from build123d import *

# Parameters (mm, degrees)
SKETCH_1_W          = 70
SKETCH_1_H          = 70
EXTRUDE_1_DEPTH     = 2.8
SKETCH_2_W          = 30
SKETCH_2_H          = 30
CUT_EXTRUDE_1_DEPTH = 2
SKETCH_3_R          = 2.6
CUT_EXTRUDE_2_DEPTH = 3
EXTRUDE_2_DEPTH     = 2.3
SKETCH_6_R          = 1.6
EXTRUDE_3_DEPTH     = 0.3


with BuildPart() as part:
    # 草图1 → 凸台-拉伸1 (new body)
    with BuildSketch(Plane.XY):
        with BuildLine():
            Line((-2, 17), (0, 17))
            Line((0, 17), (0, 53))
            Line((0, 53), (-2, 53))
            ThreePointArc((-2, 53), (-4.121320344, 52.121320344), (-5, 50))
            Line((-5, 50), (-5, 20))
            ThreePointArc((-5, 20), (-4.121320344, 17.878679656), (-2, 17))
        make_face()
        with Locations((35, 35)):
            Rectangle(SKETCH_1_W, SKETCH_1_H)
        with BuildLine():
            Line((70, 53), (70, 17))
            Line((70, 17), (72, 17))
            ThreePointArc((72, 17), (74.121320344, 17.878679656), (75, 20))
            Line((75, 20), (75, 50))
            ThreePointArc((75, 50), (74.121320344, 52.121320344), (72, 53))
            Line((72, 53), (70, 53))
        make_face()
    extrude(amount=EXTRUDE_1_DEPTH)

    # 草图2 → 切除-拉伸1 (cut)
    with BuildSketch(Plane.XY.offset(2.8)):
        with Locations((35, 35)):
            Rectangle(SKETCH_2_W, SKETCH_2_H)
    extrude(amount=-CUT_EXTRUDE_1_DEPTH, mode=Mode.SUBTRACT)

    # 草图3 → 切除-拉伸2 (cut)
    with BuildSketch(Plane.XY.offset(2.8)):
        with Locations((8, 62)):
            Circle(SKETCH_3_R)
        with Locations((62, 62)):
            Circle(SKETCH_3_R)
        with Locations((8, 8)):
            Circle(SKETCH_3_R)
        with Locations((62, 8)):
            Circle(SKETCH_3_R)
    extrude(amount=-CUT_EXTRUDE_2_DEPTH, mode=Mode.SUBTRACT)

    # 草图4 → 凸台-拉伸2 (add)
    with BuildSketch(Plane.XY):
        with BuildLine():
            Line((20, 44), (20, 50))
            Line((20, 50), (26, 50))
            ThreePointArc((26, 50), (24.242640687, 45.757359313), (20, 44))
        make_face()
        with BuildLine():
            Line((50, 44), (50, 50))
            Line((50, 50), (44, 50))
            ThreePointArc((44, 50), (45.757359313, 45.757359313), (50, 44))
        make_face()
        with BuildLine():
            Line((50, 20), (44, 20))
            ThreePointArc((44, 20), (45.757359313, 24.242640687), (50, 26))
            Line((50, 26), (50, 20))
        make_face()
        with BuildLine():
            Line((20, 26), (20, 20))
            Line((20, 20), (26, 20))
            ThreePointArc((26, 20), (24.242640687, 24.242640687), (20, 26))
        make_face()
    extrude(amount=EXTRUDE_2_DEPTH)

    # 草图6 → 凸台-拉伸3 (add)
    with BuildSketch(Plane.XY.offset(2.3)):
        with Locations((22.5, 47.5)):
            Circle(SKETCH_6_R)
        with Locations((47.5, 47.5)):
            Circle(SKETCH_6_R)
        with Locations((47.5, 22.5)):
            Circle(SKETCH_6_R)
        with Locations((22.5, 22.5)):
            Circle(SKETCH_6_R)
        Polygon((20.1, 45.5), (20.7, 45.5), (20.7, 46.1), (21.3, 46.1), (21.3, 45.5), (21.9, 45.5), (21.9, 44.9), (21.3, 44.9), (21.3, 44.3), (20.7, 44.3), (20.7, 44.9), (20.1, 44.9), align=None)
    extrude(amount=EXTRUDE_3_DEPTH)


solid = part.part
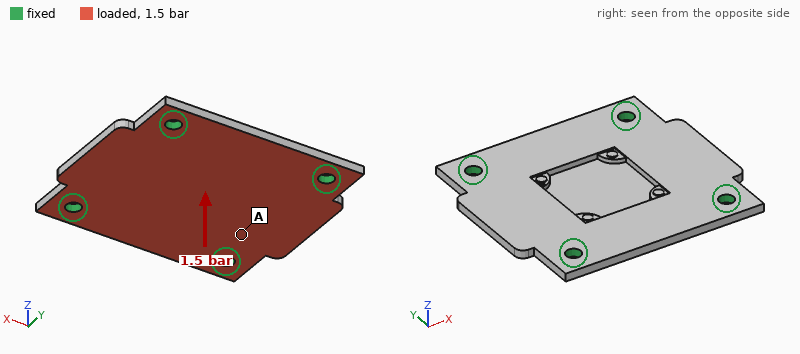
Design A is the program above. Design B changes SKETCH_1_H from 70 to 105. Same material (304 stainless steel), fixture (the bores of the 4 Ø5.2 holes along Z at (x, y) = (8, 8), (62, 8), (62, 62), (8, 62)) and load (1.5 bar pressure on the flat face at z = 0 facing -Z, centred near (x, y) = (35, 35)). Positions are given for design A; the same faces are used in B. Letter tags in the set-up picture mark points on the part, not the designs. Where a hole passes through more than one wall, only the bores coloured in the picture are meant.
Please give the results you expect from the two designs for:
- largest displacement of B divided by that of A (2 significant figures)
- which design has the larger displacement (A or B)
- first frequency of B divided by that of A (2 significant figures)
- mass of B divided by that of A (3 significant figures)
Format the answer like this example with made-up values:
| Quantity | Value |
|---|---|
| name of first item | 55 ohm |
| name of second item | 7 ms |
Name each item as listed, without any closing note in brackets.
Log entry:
| Quantity | Value |
|---|---|
| largest displacement of B divided by that of A | 0.86 |
| which design has the larger displacement | A |
| first frequency of B divided by that of A | 0.69 |
| mass of B divided by that of A | 1.53 |
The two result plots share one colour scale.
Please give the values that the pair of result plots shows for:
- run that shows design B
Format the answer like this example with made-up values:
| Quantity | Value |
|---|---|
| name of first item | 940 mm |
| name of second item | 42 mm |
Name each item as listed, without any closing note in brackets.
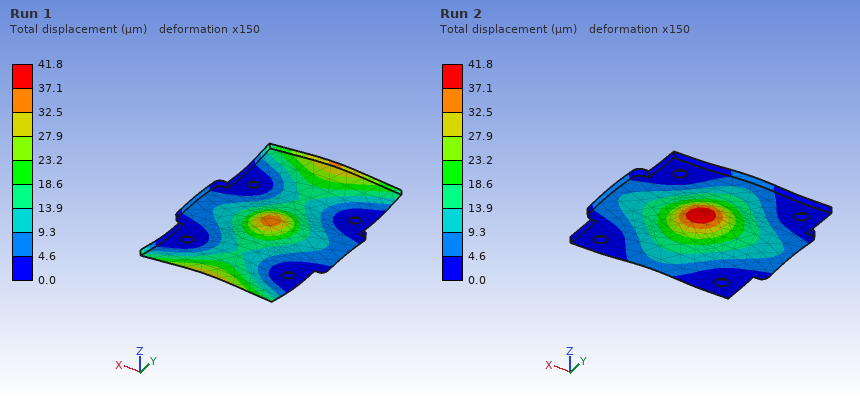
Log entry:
| Quantity | Value |
|---|---|
| run that shows design B | Run 1 |
